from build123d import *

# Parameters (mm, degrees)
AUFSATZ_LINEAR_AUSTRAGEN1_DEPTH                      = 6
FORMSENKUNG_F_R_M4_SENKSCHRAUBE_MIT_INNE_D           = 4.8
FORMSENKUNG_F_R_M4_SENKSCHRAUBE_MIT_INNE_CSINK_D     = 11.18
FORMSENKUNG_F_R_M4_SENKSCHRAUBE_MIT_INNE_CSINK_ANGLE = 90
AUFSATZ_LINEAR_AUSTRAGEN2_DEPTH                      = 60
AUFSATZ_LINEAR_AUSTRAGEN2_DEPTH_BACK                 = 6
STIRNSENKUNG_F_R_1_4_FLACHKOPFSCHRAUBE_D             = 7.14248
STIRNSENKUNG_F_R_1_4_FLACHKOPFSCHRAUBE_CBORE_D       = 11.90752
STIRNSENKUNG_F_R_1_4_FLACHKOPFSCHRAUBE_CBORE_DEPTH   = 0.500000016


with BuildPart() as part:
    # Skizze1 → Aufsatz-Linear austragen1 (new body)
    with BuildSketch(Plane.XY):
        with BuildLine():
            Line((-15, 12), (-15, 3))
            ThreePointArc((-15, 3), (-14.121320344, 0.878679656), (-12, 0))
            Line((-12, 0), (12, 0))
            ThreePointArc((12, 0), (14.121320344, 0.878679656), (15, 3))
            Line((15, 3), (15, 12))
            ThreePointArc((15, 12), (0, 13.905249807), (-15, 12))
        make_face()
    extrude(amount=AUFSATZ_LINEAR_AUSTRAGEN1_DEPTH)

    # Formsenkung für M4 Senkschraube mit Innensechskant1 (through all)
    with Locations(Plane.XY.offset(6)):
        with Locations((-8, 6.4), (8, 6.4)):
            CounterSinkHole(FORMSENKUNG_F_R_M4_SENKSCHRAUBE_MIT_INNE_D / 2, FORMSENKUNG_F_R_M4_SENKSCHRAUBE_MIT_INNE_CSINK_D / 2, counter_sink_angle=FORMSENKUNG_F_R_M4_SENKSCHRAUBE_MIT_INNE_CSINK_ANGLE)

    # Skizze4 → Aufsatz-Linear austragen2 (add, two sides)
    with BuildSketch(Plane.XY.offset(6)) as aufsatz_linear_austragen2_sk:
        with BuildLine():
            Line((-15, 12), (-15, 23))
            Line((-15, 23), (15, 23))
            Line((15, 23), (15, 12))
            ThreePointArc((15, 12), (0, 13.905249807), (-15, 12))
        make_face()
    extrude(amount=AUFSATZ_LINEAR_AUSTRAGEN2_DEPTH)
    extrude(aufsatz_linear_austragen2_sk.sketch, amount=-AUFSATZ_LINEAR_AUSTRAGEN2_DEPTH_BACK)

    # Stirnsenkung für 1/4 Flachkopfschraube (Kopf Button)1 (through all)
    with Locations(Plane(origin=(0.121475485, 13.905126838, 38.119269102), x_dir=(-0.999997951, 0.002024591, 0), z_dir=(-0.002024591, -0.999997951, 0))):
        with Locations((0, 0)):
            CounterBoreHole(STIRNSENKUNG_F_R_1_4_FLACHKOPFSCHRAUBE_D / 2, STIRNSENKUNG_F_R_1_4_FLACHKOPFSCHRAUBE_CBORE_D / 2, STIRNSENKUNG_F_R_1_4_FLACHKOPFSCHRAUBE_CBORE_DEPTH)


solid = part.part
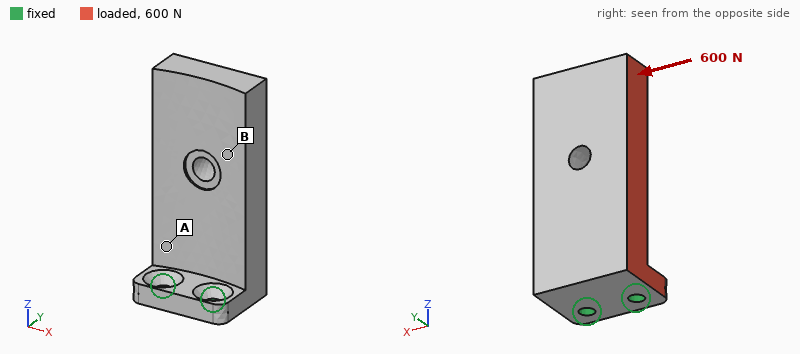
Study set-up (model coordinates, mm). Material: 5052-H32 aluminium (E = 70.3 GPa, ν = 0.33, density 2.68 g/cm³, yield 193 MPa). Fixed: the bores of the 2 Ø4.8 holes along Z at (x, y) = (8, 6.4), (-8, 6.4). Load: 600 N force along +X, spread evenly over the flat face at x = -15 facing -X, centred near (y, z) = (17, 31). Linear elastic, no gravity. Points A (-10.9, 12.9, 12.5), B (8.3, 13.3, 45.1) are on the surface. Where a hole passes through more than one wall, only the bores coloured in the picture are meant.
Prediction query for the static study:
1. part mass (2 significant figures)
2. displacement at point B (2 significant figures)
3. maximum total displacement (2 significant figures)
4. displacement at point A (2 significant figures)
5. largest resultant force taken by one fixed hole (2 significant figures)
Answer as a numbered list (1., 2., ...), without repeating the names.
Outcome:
1. 56 g
2. 63 µm
3. 96 µm
4. 21 µm
5. 1.0 kN
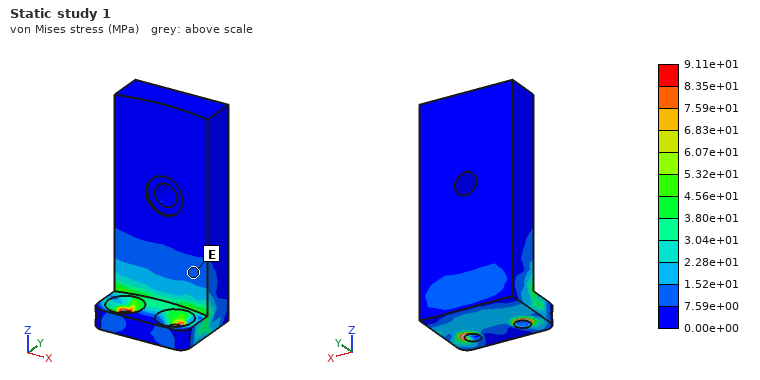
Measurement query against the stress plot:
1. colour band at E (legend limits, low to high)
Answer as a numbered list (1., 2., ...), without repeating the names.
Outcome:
1. 7.59e+00 to 1.52e+01 MPa
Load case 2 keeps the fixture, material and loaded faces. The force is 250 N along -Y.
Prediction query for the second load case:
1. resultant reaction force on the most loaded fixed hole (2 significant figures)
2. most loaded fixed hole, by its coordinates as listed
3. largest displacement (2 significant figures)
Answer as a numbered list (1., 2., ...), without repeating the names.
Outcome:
1. 320 N
2. (-8, 6.4)
3. 0.23 mm
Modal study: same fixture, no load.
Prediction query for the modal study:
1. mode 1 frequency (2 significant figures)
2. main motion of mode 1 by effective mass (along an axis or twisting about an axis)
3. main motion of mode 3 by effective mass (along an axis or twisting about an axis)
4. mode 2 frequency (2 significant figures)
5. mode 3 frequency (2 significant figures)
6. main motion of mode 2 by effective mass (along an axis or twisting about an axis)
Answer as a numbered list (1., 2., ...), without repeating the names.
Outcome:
1. 880 Hz
2. along Y
3. along Z
4. 2100 Hz
5. 6300 Hz
6. along X
